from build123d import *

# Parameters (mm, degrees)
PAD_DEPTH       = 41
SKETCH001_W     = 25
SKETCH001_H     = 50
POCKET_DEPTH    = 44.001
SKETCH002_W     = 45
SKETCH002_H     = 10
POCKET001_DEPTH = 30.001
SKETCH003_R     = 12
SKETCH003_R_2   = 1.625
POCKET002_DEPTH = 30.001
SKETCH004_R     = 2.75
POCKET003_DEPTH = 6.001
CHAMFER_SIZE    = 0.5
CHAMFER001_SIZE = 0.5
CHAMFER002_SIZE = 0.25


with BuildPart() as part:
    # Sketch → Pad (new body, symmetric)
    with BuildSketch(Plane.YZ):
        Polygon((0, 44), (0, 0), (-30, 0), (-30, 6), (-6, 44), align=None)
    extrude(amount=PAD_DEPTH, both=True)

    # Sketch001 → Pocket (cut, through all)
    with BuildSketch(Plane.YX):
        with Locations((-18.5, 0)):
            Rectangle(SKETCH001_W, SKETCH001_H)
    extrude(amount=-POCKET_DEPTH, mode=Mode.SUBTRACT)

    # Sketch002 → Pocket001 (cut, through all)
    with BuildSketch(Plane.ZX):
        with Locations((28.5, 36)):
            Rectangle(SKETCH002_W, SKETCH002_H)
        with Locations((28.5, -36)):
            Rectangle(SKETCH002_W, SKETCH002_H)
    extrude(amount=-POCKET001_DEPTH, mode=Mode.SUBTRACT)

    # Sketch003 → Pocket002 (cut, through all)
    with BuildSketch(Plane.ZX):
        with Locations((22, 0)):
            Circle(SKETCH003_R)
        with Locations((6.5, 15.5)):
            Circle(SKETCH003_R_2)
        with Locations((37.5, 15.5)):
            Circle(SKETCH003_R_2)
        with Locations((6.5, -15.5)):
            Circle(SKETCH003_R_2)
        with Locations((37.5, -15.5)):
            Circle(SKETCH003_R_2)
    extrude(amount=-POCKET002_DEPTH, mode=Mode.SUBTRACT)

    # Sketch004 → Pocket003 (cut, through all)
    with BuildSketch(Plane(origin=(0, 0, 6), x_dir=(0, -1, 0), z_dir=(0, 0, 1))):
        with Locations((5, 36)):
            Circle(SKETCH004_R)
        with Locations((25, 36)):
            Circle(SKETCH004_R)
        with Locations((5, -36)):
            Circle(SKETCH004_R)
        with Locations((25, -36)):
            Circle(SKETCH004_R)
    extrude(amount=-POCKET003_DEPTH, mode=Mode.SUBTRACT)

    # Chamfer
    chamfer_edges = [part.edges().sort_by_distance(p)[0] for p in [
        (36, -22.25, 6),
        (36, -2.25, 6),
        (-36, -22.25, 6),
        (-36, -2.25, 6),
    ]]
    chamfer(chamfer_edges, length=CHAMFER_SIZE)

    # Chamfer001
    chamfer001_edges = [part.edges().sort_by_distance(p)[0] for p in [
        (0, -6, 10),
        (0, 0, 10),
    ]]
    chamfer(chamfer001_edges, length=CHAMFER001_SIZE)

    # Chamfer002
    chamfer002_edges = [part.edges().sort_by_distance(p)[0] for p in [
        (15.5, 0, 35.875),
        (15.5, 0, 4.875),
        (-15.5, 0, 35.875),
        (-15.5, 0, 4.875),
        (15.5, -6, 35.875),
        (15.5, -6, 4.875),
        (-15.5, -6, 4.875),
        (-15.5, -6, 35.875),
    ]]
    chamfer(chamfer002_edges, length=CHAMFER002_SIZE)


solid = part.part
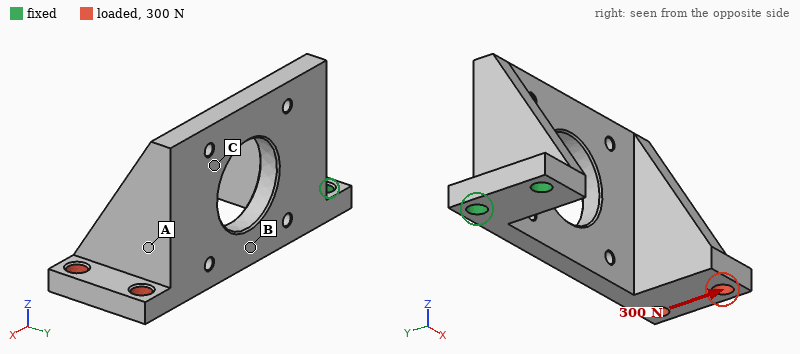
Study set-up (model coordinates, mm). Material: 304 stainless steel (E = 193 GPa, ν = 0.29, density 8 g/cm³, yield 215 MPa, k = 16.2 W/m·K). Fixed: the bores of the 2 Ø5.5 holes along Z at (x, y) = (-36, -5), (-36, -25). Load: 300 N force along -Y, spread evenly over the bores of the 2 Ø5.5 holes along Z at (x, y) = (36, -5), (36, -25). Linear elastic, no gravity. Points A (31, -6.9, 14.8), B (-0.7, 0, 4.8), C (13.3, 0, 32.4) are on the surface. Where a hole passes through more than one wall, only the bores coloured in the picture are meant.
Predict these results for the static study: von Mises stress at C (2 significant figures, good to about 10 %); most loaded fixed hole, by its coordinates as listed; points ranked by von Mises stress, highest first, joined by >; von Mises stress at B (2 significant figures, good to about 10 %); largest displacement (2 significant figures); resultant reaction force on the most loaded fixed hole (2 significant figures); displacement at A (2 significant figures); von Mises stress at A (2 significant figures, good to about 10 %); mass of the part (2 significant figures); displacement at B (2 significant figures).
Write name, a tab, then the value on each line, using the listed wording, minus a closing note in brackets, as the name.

von Mises stress at C	52 MPa
most loaded fixed hole, by its coordinates as listed	(-36, -25)
points ranked by von Mises stress, highest first, joined by >	B > C > A
von Mises stress at B	100 MPa
largest displacement	0.46 mm
resultant reaction force on the most loaded fixed hole	1.1 kN
displacement at A	0.31 mm
von Mises stress at A	19 MPa
mass of the part	190 g
displacement at B	0.093 mm
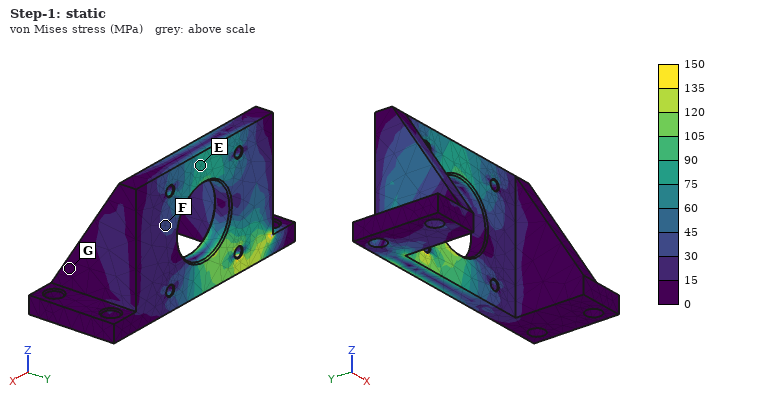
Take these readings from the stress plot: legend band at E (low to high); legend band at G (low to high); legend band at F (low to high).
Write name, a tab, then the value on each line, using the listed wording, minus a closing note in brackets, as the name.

legend band at E	75 to 90 MPa
legend band at G	0 to 15 MPa
legend band at F	30 to 45 MPa
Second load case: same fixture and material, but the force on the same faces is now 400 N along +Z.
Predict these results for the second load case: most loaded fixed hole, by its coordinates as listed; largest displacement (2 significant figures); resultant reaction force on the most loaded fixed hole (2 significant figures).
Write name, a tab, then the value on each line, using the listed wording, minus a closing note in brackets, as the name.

most loaded fixed hole, by its coordinates as listed	(-36, -25)
largest displacement	0.30 mm
resultant reaction force on the most loaded fixed hole	250 N
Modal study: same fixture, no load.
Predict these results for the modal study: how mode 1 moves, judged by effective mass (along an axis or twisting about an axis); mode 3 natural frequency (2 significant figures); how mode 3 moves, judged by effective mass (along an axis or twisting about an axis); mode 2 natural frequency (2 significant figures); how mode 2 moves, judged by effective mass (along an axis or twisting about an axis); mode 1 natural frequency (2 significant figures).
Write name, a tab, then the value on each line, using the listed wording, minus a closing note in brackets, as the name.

how mode 1 moves, judged by effective mass	along Y
mode 3 natural frequency	2000 Hz
how mode 3 moves, judged by effective mass	twisting about X
mode 2 natural frequency	750 Hz
how mode 2 moves, judged by effective mass	along Z
mode 1 natural frequency	610 Hz
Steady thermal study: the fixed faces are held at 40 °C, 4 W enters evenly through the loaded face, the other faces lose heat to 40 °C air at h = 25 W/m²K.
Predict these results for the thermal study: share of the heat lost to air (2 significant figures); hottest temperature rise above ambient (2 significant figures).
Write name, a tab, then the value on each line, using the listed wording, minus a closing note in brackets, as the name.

share of the heat lost to air	89 %
hottest temperature rise above ambient	49 K
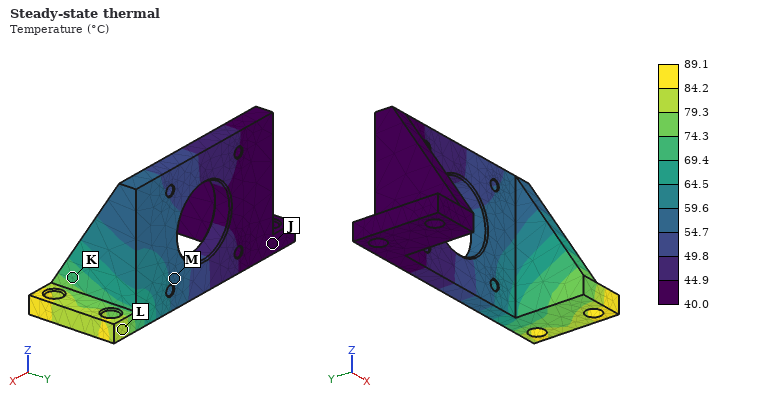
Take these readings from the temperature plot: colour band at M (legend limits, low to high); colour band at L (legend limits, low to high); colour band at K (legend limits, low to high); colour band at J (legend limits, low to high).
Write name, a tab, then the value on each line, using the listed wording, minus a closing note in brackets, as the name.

colour band at M	54.7 to 59.6 °C
colour band at L	79.3 to 84.2 °C
colour band at K	69.4 to 74.3 °C
colour band at J	40.0 to 44.9 °C
